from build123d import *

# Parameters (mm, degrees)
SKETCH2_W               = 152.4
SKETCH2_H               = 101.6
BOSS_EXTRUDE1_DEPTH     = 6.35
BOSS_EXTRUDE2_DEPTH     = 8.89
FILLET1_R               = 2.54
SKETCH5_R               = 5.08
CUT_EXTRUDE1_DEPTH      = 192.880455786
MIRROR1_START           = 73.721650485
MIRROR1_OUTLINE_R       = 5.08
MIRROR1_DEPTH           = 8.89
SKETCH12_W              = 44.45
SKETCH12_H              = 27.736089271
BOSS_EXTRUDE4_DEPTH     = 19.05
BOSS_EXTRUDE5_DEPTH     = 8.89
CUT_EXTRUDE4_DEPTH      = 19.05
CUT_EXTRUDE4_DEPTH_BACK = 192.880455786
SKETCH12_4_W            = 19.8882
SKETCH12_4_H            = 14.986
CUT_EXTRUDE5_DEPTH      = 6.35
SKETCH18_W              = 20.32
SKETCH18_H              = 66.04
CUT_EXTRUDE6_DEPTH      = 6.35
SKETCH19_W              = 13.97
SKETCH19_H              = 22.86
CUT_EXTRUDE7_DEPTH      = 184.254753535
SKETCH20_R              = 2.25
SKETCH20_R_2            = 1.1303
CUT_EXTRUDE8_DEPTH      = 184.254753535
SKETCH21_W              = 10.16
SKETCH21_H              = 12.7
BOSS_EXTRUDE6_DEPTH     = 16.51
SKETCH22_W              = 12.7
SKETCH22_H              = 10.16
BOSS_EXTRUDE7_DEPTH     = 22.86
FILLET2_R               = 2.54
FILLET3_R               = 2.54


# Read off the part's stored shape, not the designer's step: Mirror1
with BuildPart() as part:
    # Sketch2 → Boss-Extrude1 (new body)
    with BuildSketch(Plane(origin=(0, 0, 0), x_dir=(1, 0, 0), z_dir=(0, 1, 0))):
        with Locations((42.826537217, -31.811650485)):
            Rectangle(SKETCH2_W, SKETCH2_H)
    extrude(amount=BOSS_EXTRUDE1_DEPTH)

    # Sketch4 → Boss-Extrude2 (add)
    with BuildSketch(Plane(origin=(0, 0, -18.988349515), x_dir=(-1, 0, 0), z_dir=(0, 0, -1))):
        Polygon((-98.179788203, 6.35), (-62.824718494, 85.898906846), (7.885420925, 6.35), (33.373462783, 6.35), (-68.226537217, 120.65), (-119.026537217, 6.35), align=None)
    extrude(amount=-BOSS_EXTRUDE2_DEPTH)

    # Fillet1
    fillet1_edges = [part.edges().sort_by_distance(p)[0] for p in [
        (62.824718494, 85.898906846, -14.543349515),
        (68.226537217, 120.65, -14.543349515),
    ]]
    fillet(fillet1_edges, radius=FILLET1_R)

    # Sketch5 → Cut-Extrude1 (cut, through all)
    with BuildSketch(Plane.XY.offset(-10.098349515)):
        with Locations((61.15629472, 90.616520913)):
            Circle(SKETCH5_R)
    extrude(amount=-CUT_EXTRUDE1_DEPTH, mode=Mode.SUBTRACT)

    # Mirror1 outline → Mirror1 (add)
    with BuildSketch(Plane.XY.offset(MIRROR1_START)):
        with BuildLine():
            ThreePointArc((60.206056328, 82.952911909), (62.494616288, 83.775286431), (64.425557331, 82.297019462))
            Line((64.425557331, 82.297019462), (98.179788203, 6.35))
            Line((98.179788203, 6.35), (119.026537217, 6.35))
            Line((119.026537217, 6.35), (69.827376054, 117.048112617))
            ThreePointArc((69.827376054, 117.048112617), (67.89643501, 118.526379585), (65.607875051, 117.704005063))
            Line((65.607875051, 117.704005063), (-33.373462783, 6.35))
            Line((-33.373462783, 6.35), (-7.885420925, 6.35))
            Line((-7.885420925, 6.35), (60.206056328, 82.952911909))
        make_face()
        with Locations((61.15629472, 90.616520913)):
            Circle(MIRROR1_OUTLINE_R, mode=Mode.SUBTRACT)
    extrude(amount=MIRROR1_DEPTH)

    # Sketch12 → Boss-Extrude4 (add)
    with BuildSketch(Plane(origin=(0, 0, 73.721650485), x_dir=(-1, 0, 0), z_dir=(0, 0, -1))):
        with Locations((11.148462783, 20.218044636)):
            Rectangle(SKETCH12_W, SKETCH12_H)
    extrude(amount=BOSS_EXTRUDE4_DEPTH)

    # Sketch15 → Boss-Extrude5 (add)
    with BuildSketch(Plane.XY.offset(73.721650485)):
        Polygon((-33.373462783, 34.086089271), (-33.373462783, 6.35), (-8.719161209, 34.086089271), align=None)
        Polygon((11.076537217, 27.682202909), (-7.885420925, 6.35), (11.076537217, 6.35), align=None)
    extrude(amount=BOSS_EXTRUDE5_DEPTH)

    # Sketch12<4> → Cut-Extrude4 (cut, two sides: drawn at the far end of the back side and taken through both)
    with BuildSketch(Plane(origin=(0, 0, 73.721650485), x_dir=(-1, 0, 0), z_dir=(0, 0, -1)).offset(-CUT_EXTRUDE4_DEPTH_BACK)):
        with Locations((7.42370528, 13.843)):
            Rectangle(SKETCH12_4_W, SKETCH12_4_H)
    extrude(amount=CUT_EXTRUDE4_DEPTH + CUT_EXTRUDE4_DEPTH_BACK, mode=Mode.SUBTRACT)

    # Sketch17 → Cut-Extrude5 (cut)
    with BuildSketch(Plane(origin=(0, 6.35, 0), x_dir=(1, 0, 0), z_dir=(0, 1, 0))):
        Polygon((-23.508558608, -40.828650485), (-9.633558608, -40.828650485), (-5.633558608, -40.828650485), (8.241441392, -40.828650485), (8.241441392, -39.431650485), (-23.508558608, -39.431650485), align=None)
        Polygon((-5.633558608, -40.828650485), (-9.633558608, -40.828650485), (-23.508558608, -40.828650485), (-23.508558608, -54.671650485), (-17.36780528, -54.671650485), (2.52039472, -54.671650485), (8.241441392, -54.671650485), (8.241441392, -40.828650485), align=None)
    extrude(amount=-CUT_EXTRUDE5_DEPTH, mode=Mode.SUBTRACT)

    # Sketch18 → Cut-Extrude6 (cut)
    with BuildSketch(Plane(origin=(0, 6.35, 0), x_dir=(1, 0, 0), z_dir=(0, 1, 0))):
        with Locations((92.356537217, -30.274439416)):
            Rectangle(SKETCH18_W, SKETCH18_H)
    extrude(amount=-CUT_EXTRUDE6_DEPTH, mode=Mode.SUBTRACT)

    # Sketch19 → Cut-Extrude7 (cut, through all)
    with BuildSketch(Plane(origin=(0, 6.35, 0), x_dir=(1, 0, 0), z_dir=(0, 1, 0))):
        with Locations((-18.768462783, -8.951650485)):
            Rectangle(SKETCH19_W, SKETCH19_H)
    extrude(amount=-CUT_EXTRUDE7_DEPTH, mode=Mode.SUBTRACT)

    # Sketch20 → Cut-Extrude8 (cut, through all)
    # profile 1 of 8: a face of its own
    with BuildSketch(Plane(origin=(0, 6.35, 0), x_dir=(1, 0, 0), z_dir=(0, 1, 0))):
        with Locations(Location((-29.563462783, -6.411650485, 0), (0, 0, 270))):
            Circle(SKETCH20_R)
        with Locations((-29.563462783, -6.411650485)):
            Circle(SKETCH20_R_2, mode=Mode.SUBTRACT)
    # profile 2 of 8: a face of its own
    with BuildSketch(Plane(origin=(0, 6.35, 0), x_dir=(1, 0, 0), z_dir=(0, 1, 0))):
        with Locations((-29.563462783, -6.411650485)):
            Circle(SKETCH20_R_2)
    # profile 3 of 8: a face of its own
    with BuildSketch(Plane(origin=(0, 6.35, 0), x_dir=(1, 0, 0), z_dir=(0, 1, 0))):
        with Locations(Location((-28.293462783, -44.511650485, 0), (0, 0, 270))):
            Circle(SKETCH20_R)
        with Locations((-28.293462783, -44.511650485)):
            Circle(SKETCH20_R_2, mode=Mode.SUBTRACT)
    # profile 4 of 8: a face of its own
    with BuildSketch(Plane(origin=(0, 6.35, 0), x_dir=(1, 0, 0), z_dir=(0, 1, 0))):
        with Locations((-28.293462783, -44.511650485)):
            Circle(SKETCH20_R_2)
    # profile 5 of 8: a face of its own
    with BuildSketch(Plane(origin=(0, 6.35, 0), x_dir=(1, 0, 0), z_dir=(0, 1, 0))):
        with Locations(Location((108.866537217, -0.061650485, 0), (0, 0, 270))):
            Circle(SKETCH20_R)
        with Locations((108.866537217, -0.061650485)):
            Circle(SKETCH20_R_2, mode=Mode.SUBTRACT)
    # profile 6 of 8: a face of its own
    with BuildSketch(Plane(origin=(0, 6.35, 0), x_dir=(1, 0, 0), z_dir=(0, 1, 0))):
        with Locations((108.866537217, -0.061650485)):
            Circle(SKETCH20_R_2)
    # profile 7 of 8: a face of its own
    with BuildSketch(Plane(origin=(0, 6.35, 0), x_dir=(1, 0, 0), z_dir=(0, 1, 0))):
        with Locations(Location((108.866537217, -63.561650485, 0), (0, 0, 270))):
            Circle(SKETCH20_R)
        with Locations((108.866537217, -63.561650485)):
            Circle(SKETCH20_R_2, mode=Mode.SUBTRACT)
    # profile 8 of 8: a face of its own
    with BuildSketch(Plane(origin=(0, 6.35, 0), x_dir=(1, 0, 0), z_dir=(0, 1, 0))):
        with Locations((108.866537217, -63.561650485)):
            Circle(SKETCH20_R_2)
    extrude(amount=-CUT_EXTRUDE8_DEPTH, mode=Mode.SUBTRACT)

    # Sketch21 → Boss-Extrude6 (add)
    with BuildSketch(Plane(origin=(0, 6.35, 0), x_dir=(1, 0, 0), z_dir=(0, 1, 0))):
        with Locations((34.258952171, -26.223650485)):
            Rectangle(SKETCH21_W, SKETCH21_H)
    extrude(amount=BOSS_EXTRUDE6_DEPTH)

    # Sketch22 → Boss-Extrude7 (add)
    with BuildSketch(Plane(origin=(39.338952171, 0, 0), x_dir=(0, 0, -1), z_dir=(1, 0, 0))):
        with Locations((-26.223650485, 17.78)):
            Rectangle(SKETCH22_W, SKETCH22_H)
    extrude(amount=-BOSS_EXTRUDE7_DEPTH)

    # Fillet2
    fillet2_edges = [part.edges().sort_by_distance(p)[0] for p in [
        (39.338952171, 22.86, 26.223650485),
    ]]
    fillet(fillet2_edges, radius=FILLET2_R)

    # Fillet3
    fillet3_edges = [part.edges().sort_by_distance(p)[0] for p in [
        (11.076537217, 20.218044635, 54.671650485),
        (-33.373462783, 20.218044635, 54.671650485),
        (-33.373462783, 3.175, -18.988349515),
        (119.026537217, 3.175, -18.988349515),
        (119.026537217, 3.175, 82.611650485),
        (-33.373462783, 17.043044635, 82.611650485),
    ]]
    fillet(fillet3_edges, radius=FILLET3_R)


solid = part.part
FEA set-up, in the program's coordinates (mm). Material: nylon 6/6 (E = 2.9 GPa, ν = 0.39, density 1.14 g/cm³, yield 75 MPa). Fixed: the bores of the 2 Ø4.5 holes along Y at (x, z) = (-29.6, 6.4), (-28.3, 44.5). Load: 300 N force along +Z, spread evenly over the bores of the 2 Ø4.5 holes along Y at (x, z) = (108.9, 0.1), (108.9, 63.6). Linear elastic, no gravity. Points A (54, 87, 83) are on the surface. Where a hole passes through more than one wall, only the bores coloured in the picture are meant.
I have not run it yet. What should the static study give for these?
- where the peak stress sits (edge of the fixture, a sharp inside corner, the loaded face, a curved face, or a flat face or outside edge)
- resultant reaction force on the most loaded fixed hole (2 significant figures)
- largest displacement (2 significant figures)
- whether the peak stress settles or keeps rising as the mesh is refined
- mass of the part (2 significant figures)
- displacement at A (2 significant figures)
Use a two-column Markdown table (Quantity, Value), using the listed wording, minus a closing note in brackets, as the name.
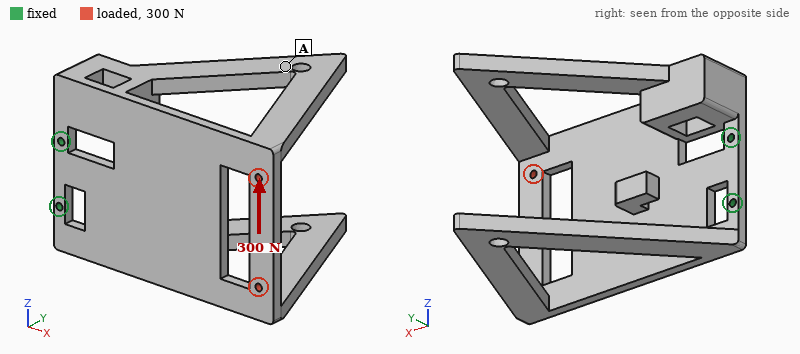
| Quantity | Value |
|---|---|
| where the peak stress sits | edge of the fixture |
| resultant reaction force on the most loaded fixed hole | 970 N |
| largest displacement | 2.5 mm |
| whether the peak stress settles or keeps rising as the mesh is refined | keeps rising |
| mass of the part | 210 g |
| displacement at A | 1.5 mm |
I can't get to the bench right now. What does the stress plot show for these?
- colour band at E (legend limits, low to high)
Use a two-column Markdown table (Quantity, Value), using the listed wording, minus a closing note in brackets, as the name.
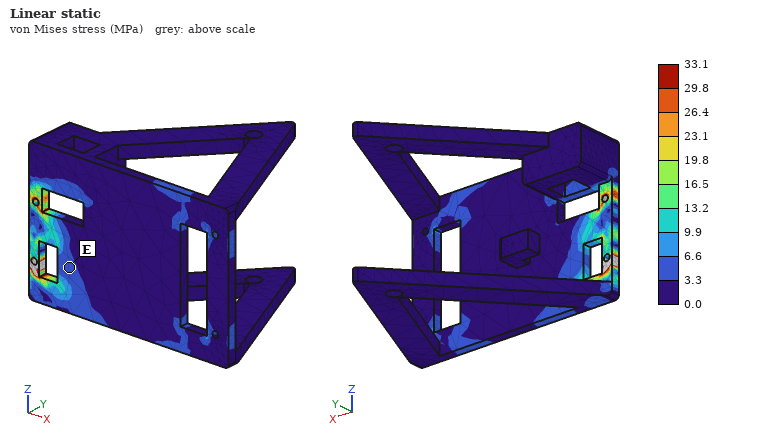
| Quantity | Value |
|---|---|
| colour band at E | 3.3 to 6.6 MPa |
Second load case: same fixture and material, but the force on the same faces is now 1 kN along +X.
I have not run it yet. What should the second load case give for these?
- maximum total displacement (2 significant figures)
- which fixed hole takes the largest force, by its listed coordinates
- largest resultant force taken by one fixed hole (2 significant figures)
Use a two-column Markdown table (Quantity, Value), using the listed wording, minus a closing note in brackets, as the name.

| Quantity | Value |
|---|---|
| maximum total displacement | 0.42 mm |
| which fixed hole takes the largest force, by its listed coordinates | (-28.3, 44.5) |
| largest resultant force taken by one fixed hole | 680 N |
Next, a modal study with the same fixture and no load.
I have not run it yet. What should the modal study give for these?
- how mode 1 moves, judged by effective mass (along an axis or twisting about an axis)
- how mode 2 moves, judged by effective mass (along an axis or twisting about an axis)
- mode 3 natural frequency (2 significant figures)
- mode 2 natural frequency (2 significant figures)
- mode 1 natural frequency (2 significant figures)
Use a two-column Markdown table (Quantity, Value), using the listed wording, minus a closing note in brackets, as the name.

| Quantity | Value |
|---|---|
| how mode 1 moves, judged by effective mass | along Y |
| how mode 2 moves, judged by effective mass | along Z |
| mode 3 natural frequency | 120 Hz |
| mode 2 natural frequency | 74 Hz |
| mode 1 natural frequency | 43 Hz |
